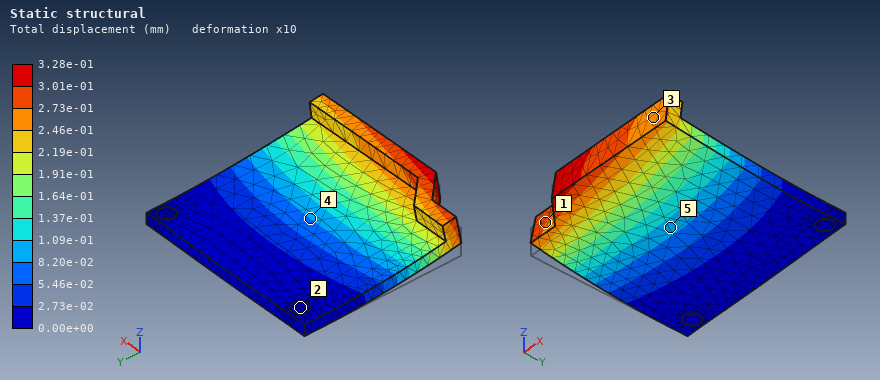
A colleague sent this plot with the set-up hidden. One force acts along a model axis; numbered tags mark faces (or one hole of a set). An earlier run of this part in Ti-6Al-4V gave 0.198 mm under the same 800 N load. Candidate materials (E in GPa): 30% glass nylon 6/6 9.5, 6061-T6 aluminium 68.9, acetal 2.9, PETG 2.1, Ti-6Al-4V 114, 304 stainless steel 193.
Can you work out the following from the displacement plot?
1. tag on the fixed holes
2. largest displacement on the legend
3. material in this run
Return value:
2
3.28e-01 mm
6061-T6 aluminium
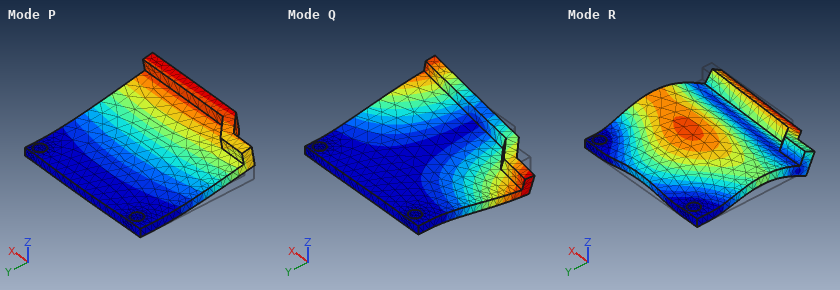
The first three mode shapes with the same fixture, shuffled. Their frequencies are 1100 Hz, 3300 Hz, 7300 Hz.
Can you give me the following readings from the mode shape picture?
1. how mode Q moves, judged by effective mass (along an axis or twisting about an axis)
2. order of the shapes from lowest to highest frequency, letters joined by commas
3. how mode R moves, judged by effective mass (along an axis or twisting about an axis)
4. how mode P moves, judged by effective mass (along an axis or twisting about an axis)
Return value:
twisting about Y
P, Q, R
along Z
along Z
